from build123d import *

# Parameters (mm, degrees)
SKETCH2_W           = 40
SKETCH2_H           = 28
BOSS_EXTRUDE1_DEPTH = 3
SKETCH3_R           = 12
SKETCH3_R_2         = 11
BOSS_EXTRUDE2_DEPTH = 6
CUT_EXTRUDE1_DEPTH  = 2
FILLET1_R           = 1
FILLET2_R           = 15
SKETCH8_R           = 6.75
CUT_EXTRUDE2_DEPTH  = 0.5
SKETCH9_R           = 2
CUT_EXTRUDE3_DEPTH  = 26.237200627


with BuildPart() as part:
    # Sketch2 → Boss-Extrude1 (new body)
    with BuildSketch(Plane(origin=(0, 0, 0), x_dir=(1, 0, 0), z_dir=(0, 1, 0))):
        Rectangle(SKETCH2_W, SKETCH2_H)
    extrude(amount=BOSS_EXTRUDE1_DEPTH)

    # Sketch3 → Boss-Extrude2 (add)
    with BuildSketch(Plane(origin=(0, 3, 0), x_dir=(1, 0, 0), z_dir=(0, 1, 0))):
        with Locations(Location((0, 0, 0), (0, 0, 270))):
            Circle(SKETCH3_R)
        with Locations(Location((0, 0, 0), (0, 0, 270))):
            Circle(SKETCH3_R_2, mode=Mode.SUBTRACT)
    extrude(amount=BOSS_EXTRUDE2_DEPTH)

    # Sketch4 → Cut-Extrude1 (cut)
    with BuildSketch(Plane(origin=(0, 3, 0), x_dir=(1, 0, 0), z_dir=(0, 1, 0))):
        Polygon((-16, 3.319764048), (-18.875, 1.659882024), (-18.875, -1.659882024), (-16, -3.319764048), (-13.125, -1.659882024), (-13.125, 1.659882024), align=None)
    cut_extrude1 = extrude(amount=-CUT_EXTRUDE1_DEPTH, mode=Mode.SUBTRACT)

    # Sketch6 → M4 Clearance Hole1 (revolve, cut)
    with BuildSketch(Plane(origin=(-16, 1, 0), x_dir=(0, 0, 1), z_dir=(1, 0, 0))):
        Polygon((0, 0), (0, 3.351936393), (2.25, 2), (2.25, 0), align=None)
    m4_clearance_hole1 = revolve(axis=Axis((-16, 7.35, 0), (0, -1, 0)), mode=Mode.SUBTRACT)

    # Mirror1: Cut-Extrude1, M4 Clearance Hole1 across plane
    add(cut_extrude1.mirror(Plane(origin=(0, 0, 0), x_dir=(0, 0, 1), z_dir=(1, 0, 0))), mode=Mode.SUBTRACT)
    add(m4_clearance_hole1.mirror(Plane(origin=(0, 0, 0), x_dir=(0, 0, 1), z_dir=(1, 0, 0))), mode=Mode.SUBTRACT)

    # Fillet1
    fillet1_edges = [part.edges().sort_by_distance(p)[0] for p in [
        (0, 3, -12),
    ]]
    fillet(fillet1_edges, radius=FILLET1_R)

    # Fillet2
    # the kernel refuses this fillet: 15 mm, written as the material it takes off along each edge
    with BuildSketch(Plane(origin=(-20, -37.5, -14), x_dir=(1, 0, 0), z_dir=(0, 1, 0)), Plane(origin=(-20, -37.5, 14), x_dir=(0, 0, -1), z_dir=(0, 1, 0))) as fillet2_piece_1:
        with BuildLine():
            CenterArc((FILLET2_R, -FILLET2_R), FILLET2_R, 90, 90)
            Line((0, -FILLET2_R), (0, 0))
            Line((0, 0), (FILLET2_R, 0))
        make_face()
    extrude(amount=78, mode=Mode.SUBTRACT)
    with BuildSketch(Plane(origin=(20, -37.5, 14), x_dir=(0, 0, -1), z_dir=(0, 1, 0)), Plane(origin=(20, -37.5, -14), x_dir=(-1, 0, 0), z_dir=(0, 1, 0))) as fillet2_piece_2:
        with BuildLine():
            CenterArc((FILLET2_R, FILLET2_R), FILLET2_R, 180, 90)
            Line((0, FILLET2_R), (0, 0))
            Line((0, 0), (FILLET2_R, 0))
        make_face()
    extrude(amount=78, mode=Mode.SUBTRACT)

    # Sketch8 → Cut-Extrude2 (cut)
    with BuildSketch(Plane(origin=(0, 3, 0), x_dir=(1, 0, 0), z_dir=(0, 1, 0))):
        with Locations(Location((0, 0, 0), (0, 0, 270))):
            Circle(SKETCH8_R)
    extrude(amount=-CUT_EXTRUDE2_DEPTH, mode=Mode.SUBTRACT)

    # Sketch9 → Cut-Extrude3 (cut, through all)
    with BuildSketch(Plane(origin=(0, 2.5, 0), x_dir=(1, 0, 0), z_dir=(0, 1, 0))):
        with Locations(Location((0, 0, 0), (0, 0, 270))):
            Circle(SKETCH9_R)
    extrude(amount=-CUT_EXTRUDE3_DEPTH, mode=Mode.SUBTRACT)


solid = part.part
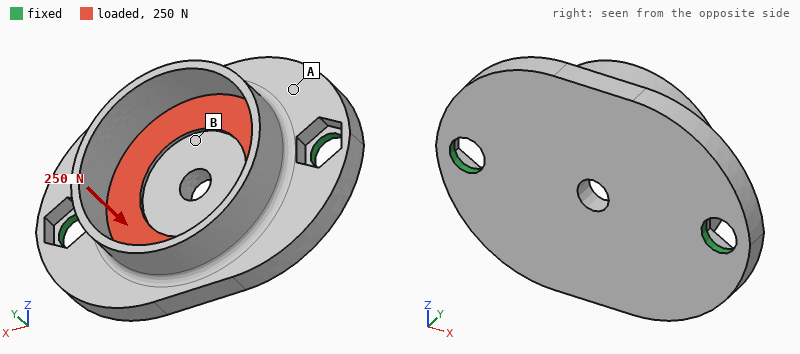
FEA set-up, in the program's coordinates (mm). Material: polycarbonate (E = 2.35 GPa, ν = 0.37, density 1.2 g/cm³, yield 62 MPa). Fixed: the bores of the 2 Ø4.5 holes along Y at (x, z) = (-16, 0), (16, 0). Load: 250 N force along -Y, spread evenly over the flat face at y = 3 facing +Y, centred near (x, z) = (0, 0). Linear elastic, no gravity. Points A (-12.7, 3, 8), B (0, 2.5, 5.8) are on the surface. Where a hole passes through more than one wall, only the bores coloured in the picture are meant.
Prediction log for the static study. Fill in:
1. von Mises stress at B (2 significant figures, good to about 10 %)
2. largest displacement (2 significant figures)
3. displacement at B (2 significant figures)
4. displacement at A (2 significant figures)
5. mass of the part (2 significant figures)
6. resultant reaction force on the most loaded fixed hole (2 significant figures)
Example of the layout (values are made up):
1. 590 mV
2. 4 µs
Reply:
1. 12 MPa
2. 0.54 mm
3. 0.35 mm
4. 0.15 mm
5. 3.6 g
6. 190 N
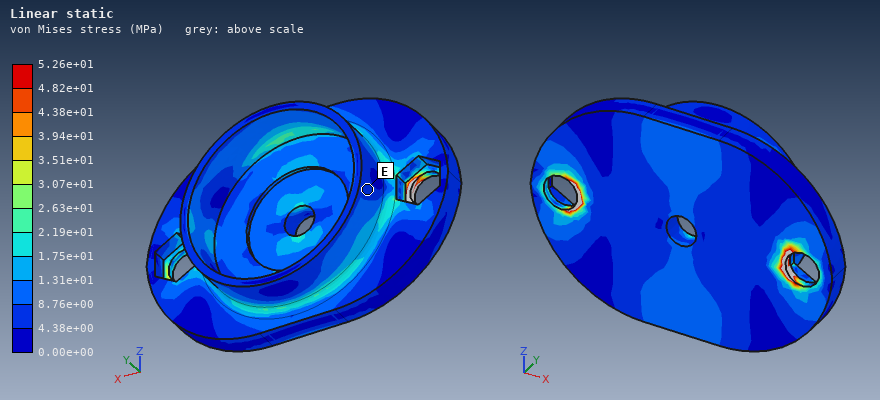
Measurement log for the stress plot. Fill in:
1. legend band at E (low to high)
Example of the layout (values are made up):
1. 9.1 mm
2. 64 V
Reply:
1. 4.38e+00 to 8.76e+00 MPa
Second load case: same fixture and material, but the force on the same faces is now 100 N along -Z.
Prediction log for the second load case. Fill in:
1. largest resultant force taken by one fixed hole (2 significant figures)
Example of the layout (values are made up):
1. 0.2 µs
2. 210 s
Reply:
1. 50 N
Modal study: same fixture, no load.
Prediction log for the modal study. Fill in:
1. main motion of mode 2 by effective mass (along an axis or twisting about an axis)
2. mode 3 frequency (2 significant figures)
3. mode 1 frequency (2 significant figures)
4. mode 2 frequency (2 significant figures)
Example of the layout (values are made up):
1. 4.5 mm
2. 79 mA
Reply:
1. along Y
2. 4600 Hz
3. 1600 Hz
4. 2500 Hz
